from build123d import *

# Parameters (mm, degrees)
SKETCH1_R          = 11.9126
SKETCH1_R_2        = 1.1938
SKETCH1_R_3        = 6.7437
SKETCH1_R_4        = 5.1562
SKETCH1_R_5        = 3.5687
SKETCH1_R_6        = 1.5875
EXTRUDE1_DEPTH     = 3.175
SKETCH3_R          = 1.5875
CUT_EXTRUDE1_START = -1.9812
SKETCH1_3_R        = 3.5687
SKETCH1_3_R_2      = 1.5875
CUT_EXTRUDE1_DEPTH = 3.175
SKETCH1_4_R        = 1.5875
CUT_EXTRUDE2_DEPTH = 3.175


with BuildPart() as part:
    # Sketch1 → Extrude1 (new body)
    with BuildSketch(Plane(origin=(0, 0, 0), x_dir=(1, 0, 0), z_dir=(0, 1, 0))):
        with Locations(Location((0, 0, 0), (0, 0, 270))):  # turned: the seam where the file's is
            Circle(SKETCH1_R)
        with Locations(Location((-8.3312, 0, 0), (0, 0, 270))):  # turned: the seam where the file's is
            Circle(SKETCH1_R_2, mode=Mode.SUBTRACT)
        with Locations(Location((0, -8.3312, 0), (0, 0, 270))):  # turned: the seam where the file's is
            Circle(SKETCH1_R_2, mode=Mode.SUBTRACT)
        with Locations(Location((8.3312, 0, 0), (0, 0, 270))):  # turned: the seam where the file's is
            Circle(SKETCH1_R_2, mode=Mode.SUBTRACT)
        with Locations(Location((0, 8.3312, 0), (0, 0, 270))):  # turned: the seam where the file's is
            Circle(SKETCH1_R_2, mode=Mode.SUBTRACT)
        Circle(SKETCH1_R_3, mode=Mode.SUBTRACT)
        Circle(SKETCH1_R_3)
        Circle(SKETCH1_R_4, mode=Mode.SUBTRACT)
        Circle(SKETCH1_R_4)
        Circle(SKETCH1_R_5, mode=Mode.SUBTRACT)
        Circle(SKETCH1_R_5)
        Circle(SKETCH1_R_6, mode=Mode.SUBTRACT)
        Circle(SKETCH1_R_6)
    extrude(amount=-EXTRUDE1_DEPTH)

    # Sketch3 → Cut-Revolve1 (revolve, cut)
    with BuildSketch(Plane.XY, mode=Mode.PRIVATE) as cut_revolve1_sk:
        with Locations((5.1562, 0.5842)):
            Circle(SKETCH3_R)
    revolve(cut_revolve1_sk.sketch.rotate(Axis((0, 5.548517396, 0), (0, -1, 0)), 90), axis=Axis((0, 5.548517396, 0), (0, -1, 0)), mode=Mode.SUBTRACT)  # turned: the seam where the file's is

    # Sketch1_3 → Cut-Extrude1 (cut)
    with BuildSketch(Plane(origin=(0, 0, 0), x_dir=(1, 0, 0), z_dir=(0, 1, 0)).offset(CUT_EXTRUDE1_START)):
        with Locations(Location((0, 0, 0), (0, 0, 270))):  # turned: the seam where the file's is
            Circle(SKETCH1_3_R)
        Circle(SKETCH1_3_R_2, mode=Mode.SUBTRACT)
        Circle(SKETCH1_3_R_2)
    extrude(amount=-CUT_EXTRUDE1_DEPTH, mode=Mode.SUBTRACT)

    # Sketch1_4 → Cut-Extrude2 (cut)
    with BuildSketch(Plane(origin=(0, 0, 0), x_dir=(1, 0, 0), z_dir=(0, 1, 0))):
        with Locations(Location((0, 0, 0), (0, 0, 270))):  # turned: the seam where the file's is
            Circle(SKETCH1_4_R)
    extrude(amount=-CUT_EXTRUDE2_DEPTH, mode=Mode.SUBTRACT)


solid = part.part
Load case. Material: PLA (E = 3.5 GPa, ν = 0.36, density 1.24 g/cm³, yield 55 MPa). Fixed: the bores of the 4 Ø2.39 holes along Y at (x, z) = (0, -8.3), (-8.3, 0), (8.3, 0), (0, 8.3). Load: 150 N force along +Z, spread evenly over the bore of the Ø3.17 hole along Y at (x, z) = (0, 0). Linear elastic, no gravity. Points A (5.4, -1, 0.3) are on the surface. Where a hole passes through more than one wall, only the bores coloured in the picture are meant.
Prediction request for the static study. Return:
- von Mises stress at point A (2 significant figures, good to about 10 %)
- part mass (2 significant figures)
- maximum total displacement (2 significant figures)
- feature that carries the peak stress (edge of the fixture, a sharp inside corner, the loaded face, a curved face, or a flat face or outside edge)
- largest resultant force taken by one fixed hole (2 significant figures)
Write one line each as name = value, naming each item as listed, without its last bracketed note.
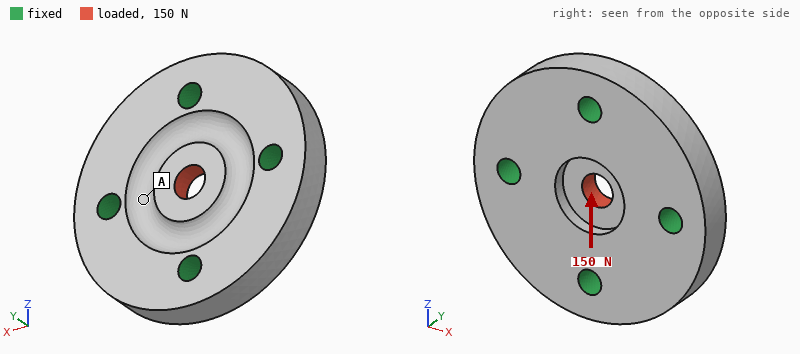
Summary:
von Mises stress at point A = 1.8 MPa
part mass = 1.5 g
maximum total displacement = 14 µm
feature that carries the peak stress = the loaded face
largest resultant force taken by one fixed hole = 49 N
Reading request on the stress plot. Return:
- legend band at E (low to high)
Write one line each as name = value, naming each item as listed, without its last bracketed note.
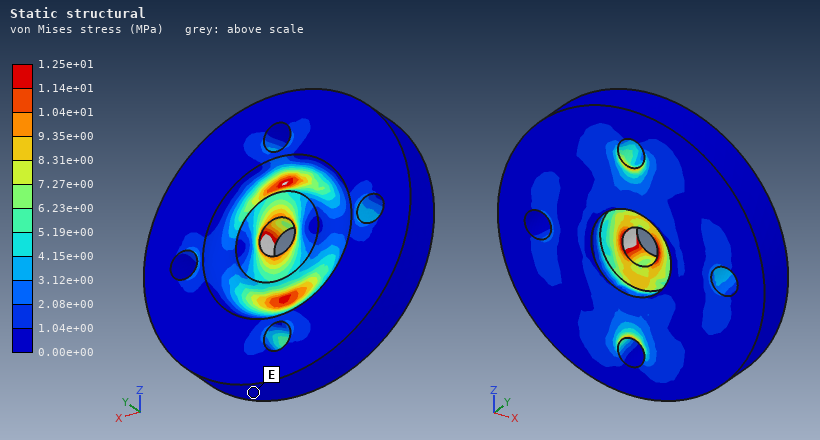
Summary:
legend band at E = 0.00e+00 to 1.04e+00 MPa
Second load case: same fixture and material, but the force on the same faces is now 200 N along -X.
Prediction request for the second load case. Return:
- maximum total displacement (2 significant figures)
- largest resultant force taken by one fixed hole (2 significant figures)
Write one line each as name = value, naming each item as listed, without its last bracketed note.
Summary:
maximum total displacement = 19 µm
largest resultant force taken by one fixed hole = 66 N
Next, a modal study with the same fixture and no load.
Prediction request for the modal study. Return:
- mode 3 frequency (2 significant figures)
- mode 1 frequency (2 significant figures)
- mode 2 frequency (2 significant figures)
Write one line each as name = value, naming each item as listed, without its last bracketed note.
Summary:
mode 3 frequency = 21 kHz
mode 1 frequency = 20 kHz
mode 2 frequency = 21 kHz
